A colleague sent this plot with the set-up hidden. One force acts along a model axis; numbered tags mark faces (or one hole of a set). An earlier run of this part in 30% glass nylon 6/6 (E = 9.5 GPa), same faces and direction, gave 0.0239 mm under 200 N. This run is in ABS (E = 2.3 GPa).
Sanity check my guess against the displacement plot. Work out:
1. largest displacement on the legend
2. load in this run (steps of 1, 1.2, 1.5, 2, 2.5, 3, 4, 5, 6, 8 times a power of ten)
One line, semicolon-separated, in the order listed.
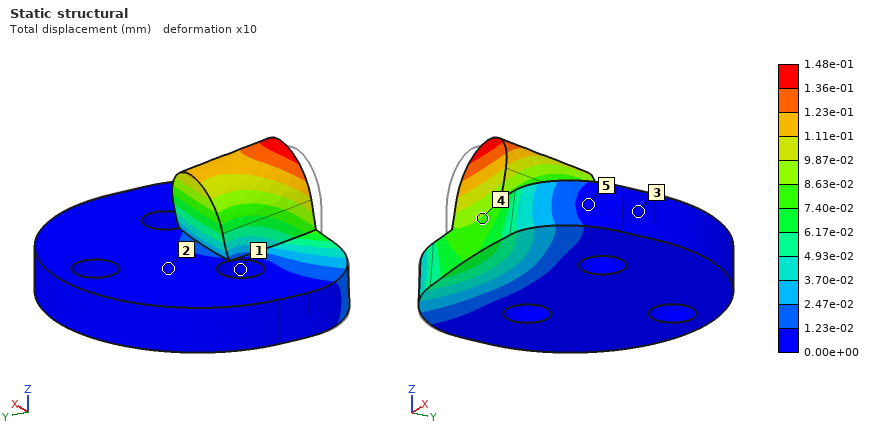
1.48e-01 mm; 300 N
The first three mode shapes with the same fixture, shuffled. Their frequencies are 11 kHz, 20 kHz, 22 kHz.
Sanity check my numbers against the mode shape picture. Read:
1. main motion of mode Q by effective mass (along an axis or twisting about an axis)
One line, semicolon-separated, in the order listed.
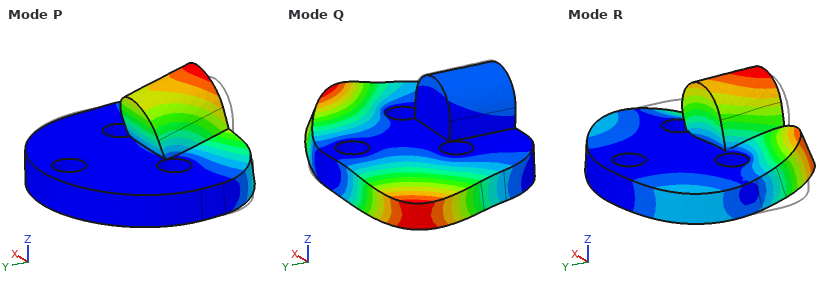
twisting about Y
